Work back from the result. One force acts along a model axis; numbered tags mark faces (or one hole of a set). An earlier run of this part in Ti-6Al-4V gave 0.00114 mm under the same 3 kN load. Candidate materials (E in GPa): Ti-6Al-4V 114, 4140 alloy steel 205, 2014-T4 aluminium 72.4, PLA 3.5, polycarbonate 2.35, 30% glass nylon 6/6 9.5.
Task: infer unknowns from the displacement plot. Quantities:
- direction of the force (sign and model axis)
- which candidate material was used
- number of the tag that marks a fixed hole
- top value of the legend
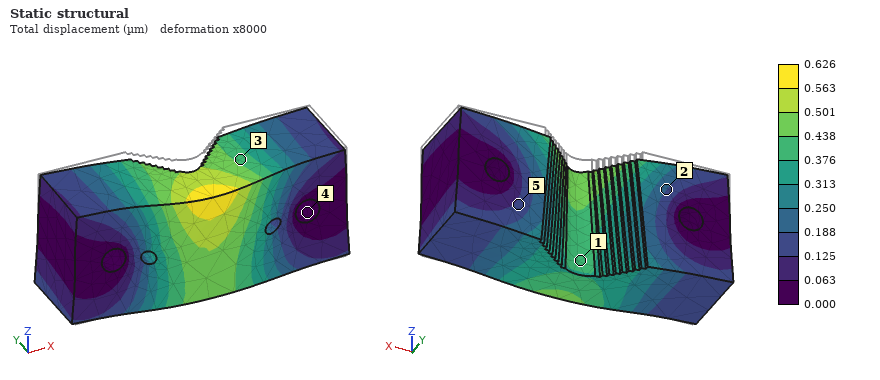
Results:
-Z
4140 alloy steel
4
0.626 µm
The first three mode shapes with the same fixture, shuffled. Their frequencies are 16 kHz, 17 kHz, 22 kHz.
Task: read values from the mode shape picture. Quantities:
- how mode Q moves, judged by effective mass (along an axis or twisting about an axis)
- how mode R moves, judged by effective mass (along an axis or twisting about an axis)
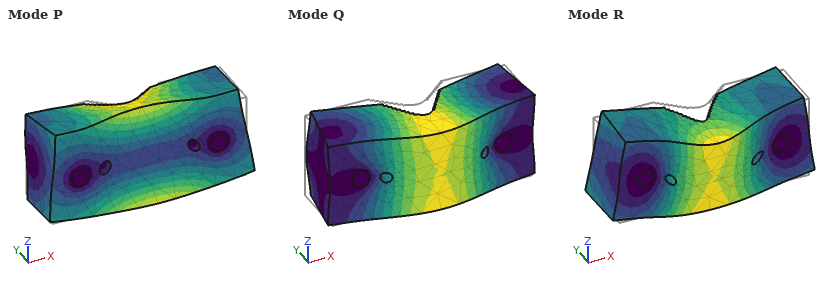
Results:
along Y
along Z
